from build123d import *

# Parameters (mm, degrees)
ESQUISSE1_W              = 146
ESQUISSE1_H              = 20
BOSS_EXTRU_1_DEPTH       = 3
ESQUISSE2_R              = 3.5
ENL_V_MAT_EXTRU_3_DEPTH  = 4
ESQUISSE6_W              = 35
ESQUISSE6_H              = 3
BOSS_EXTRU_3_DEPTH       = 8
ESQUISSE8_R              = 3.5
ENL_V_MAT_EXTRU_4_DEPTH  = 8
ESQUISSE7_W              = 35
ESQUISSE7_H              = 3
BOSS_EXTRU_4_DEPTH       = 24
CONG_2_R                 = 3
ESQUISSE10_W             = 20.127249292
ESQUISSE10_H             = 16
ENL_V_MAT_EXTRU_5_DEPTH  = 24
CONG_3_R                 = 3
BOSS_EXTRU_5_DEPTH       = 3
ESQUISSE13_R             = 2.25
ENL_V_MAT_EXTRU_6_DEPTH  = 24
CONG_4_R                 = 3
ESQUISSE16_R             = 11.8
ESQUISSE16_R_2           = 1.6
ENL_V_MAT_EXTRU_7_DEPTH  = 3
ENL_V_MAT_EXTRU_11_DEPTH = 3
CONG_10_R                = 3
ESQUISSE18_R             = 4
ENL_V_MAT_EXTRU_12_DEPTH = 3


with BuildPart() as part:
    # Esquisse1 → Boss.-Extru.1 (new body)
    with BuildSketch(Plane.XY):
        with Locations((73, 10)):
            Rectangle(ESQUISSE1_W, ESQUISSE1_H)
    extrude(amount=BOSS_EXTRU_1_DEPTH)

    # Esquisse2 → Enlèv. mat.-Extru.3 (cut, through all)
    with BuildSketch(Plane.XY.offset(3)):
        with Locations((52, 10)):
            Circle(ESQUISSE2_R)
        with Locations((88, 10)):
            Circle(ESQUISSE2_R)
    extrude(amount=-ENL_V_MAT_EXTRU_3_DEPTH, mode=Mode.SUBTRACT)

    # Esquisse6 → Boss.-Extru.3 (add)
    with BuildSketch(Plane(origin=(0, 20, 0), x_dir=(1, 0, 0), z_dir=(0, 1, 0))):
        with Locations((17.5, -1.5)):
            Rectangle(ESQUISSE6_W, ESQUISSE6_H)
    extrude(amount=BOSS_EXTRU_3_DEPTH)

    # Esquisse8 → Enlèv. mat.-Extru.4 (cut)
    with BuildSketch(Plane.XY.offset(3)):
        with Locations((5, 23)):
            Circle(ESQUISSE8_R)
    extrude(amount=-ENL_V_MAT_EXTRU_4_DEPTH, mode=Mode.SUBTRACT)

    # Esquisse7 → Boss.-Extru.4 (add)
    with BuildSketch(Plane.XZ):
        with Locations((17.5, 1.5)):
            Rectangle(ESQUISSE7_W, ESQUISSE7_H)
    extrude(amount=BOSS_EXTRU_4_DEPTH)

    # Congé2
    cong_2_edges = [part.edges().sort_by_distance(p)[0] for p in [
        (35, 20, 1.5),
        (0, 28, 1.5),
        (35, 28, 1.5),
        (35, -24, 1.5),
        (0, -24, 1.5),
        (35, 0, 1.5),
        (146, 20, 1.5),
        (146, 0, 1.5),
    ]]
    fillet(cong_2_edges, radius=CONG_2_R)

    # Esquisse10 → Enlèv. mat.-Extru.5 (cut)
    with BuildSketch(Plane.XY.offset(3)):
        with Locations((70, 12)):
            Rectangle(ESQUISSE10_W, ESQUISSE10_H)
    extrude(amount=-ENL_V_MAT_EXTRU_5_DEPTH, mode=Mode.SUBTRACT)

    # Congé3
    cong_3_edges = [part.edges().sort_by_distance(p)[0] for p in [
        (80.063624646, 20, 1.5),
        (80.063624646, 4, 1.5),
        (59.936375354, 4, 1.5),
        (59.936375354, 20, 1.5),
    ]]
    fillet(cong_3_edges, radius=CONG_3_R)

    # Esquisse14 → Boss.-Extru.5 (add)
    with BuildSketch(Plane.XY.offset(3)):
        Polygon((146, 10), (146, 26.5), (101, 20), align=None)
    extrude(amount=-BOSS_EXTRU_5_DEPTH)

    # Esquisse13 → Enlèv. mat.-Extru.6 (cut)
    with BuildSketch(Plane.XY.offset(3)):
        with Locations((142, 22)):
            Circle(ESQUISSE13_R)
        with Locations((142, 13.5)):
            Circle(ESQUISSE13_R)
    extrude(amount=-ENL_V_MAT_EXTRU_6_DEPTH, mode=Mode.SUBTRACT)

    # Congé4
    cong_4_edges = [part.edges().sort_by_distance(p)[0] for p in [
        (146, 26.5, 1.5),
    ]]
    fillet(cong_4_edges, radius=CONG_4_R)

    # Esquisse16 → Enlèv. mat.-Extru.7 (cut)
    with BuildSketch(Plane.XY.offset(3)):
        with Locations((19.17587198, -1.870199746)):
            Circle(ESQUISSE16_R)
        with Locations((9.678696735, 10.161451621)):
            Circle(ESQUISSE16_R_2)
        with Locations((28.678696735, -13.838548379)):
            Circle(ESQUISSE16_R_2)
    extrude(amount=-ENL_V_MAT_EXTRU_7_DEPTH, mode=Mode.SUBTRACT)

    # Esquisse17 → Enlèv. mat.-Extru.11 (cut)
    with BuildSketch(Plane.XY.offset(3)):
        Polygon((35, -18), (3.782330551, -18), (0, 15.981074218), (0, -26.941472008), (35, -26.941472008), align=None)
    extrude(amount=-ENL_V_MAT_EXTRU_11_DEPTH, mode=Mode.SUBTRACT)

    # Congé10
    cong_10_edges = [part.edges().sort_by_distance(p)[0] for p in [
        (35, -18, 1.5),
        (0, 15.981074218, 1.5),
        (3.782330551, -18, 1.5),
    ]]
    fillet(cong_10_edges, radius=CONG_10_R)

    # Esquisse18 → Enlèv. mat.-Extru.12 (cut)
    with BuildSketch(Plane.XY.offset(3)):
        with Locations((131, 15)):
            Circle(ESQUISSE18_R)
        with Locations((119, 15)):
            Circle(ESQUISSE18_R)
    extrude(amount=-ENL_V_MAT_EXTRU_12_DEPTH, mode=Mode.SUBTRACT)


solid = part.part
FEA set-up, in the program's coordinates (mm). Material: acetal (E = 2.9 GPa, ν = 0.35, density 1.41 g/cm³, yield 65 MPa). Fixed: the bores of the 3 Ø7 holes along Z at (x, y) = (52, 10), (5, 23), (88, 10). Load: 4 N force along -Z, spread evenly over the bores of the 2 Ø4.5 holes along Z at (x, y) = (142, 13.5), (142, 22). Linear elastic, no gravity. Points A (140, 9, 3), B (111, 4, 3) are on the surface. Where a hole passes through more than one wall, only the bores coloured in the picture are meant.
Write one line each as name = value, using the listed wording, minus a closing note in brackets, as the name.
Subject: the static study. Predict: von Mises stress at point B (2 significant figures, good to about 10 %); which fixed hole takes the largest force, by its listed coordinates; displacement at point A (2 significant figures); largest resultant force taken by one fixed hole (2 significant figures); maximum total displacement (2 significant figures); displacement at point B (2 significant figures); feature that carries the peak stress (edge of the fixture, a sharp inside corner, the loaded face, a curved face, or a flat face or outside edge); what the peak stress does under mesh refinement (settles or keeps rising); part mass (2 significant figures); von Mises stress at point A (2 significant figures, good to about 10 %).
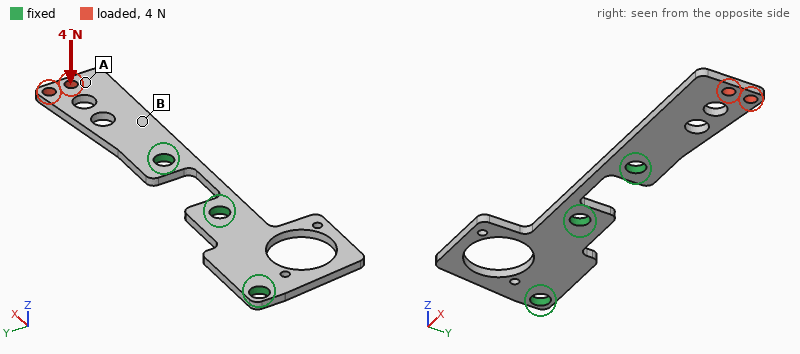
von Mises stress at point B = 4.2 MPa
which fixed hole takes the largest force, by its listed coordinates = (88, 10)
displacement at point A = 1.3 mm
largest resultant force taken by one fixed hole = 4.0 N
maximum total displacement = 1.7 mm
displacement at point B = 0.27 mm
feature that carries the peak stress = edge of the fixture
what the peak stress does under mesh refinement = keeps rising
part mass = 12 g
von Mises stress at point A = 0.83 MPa
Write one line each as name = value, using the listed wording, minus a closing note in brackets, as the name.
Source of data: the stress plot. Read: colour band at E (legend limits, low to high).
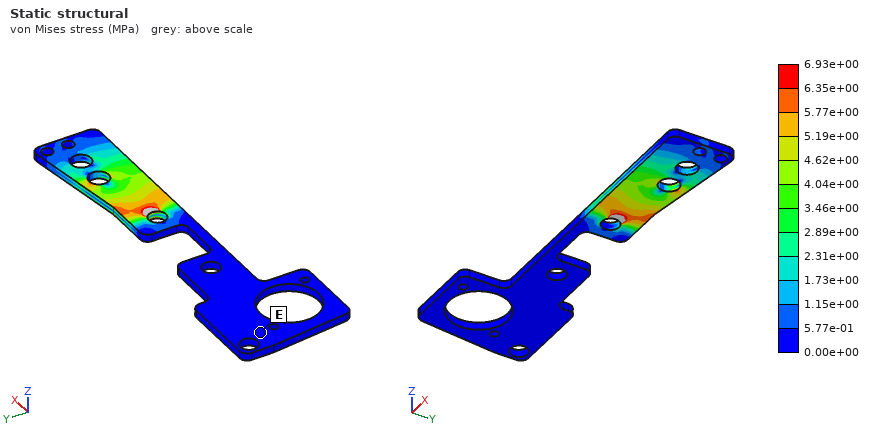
colour band at E = 0.00e+00 to 5.77e-01 MPa
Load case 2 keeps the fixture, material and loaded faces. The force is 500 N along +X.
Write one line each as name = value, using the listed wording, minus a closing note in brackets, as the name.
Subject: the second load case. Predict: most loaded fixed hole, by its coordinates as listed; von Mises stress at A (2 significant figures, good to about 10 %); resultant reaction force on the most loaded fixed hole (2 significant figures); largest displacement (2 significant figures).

most loaded fixed hole, by its coordinates as listed = (88, 10)
von Mises stress at A = 6.7 MPa
resultant reaction force on the most loaded fixed hole = 530 N
largest displacement = 1.5 mm
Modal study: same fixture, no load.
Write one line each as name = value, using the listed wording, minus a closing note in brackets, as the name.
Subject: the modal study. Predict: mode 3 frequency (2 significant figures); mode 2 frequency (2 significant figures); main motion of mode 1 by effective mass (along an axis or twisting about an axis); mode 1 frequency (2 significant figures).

mode 3 frequency = 890 Hz
mode 2 frequency = 550 Hz
main motion of mode 1 by effective mass = along Z
mode 1 frequency = 220 Hz
